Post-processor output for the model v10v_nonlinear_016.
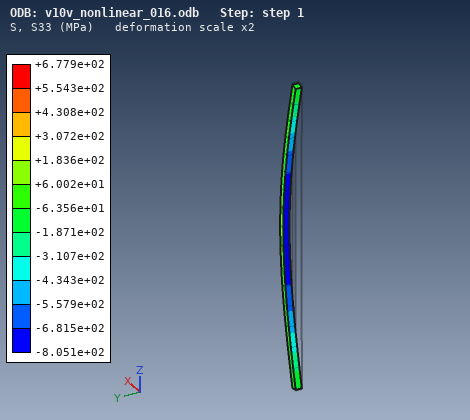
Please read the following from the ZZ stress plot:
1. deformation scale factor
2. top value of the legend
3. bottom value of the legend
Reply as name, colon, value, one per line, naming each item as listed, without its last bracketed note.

deformation scale factor: 2
top value of the legend: +6.779e+02 MPa
bottom value of the legend: -8.051e+02 MPa
